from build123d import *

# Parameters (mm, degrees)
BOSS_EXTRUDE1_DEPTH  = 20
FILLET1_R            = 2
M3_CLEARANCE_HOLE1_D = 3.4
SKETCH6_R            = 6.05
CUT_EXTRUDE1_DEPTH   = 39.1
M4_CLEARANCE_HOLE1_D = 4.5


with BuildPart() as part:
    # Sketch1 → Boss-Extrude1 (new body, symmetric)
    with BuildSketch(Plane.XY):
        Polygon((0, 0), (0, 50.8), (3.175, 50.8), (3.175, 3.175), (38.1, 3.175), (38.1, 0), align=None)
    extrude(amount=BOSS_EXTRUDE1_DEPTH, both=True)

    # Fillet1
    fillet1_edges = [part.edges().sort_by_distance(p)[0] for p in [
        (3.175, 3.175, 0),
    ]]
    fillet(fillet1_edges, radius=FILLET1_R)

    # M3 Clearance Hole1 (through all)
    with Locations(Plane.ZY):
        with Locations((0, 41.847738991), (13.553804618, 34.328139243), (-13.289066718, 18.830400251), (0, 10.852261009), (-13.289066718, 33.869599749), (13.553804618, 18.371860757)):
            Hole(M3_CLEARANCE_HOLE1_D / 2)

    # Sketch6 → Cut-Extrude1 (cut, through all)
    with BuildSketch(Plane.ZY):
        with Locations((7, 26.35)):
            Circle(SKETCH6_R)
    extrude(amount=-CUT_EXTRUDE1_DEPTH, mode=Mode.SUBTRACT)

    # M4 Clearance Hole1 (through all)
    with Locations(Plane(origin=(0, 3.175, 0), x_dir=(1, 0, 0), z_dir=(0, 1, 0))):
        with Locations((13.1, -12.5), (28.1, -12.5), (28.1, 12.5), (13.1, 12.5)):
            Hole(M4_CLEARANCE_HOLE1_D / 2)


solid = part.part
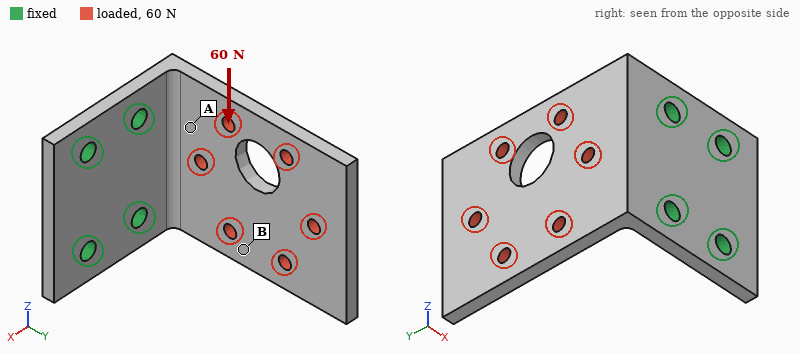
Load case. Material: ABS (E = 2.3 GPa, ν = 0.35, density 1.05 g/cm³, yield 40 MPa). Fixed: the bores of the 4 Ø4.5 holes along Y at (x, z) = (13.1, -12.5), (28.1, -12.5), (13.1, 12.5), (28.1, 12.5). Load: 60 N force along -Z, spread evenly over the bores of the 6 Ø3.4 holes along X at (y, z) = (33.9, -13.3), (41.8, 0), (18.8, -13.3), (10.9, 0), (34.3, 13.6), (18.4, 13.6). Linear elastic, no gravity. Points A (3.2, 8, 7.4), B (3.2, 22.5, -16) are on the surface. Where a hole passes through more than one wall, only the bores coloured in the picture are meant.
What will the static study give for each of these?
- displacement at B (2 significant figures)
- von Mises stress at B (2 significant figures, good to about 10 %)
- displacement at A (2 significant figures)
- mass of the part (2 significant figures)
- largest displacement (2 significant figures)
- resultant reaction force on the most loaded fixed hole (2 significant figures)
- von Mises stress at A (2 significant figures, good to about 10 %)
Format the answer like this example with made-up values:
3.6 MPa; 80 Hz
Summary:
0.29 mm; 1.7 MPa; 0.095 mm; 11 g; 0.56 mm; 67 N; 4.2 MPa
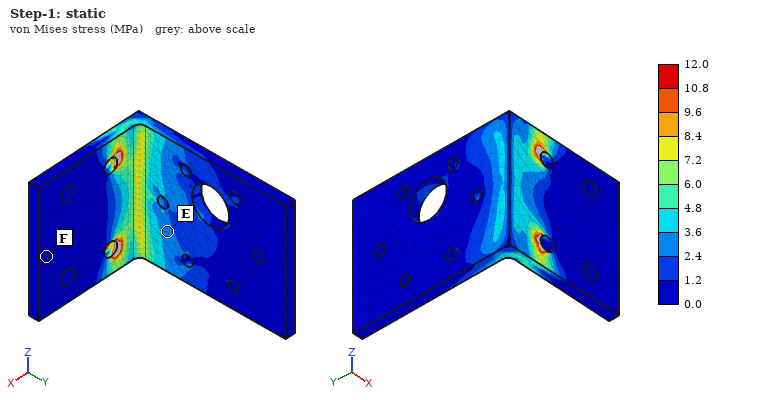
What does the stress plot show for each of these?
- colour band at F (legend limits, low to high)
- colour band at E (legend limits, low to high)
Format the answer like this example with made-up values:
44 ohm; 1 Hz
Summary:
0.0 to 1.2 MPa; 2.4 to 3.6 MPa
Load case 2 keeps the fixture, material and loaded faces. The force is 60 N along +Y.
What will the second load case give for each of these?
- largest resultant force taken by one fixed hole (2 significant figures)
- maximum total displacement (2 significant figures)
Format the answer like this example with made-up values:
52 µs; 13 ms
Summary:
35 N; 0.69 mm
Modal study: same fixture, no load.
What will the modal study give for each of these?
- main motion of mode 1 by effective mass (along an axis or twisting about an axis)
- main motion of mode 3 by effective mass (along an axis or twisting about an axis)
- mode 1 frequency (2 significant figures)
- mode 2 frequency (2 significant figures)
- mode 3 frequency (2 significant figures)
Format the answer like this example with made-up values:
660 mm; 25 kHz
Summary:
along X; along Z; 250 Hz; 700 Hz; 960 Hz
